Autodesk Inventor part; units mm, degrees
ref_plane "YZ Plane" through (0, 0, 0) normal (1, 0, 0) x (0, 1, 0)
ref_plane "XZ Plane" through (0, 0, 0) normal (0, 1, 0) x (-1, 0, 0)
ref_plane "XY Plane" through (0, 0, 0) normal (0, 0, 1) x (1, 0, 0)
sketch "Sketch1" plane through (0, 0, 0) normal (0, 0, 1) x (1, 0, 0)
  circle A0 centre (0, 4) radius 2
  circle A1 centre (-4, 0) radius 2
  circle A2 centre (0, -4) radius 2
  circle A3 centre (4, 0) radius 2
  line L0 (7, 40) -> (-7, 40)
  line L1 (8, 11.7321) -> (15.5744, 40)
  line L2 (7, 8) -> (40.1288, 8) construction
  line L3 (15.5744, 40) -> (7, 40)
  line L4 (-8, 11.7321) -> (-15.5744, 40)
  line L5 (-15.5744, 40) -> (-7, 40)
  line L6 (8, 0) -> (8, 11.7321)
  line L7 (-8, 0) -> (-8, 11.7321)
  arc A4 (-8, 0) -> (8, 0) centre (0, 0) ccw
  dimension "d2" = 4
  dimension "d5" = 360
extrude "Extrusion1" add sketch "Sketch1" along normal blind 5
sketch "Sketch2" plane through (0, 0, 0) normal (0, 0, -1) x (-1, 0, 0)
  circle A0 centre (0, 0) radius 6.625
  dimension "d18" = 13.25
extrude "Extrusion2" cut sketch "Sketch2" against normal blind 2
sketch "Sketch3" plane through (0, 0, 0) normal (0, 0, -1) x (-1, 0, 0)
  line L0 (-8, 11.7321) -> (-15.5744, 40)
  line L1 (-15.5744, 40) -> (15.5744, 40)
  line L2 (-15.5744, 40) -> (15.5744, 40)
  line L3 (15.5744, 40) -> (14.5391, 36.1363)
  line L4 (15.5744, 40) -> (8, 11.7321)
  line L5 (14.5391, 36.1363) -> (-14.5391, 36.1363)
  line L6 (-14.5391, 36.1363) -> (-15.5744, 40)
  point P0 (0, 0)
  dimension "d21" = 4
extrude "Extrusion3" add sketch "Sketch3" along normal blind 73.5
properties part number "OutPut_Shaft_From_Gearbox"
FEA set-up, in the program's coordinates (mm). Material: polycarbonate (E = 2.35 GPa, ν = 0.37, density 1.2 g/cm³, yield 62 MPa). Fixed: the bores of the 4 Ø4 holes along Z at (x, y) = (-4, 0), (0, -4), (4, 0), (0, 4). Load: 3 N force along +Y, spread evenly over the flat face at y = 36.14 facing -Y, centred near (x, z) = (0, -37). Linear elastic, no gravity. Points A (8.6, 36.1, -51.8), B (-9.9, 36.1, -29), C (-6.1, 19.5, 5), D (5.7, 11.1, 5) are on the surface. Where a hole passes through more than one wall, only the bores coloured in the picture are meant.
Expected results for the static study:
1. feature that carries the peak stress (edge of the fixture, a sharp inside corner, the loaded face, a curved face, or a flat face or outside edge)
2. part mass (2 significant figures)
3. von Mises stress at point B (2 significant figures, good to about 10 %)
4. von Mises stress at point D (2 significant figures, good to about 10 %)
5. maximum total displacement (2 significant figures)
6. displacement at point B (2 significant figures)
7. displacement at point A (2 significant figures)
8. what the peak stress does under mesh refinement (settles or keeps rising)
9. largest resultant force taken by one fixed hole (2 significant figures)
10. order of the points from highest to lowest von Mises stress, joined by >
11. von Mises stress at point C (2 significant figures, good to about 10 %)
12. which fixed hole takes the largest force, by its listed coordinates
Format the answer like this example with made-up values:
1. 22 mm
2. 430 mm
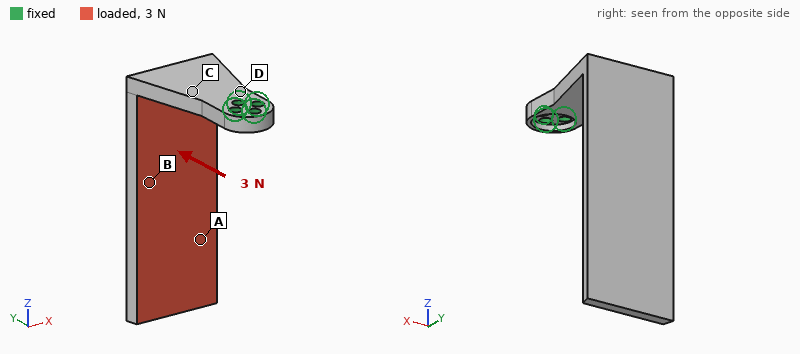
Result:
1. edge of the fixture
2. 15 g
3. 0.55 MPa
4. 1.7 MPa
5. 1.2 mm
6. 0.43 mm
7. 0.78 mm
8. keeps rising
9. 12 N
10. D > C > B > A
11. 1.4 MPa
12. (0, 4)
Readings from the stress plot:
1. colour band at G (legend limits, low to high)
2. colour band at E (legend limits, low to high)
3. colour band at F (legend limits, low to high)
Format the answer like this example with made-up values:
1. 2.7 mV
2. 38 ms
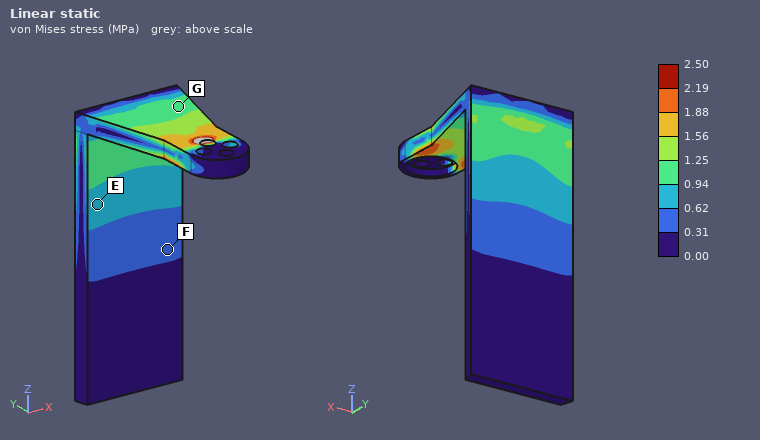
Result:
1. 0.94 to 1.25 MPa
2. 0.62 to 0.94 MPa
3. 0.31 to 0.62 MPa
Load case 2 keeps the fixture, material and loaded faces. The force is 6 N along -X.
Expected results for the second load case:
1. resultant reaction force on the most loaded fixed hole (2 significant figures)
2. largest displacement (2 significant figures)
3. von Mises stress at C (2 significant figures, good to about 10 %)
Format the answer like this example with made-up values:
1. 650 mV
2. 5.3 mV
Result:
1. 18 N
2. 1.1 mm
3. 2.5 MPa
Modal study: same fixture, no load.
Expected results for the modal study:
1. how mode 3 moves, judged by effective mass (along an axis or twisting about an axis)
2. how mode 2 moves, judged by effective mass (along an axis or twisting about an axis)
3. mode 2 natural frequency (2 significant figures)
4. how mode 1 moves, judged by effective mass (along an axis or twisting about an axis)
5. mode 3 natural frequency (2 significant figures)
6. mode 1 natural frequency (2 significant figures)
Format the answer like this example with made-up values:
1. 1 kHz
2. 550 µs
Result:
1. along Z
2. along X
3. 140 Hz
4. along Y
5. 320 Hz
6. 95 Hz
